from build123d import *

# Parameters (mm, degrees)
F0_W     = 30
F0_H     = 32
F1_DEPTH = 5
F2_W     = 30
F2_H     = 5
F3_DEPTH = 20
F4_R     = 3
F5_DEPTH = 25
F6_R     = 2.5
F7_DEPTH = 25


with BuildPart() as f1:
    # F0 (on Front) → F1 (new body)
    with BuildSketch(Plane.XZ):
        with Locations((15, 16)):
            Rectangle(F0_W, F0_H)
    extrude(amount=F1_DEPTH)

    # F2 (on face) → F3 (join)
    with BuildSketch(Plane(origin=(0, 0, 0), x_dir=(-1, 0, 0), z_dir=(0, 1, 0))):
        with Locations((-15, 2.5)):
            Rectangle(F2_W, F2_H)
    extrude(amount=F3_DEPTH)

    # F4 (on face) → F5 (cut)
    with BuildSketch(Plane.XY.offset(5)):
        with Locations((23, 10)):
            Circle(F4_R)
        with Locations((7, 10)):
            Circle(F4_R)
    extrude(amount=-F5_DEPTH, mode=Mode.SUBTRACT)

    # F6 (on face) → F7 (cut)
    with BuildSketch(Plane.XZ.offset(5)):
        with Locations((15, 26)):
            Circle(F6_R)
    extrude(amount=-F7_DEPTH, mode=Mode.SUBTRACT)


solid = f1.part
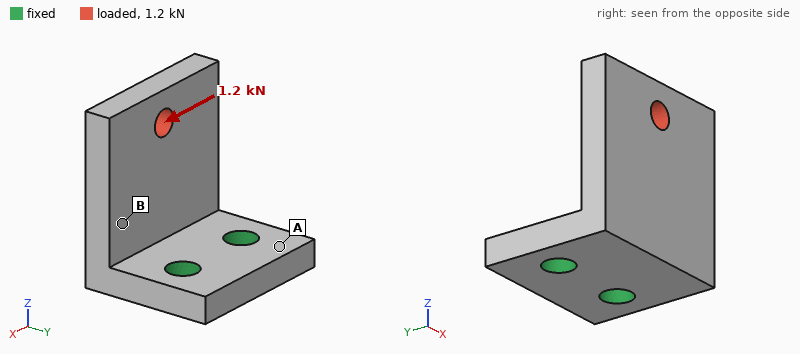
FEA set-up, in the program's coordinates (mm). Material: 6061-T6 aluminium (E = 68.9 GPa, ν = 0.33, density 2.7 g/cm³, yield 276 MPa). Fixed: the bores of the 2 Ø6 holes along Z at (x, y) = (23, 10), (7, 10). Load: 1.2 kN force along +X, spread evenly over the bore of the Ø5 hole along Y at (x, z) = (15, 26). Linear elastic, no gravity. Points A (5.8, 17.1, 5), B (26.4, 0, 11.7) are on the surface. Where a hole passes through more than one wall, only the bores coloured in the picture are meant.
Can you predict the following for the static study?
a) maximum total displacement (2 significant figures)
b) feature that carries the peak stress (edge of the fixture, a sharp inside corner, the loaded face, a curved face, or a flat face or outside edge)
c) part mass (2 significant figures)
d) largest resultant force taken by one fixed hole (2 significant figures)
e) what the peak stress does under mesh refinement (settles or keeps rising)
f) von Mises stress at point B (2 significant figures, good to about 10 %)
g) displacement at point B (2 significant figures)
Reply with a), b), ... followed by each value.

a) 0.14 mm
b) edge of the fixture
c) 20 g
d) 1.6 kN
e) keeps rising
f) 50 MPa
g) 0.057 mm
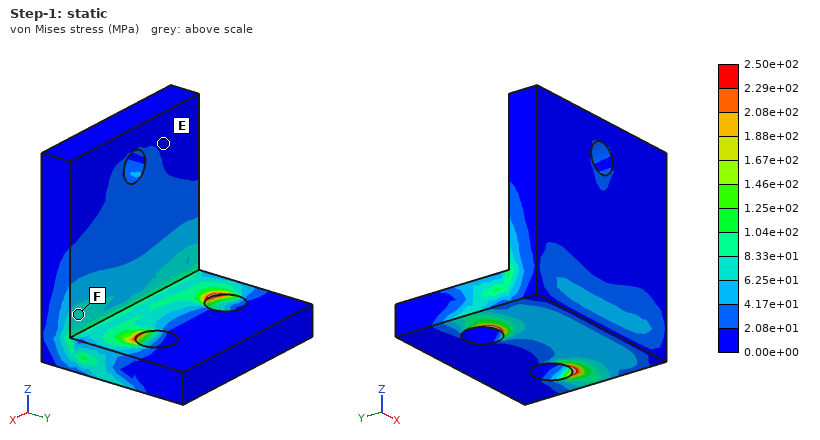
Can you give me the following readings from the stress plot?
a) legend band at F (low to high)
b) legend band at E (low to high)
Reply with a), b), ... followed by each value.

a) 6.25e+01 to 8.33e+01 MPa
b) 0.00e+00 to 2.08e+01 MPa
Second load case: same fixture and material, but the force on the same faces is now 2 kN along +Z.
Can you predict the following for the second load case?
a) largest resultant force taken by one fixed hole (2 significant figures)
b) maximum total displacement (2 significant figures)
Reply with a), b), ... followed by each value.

a) 1.0 kN
b) 0.17 mm
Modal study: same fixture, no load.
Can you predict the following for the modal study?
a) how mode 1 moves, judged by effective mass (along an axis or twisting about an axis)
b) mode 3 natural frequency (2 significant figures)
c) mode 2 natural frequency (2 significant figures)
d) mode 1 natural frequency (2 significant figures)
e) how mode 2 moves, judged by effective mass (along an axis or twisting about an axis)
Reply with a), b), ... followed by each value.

a) along Y
b) 10000 Hz
c) 6400 Hz
d) 3200 Hz
e) along X
